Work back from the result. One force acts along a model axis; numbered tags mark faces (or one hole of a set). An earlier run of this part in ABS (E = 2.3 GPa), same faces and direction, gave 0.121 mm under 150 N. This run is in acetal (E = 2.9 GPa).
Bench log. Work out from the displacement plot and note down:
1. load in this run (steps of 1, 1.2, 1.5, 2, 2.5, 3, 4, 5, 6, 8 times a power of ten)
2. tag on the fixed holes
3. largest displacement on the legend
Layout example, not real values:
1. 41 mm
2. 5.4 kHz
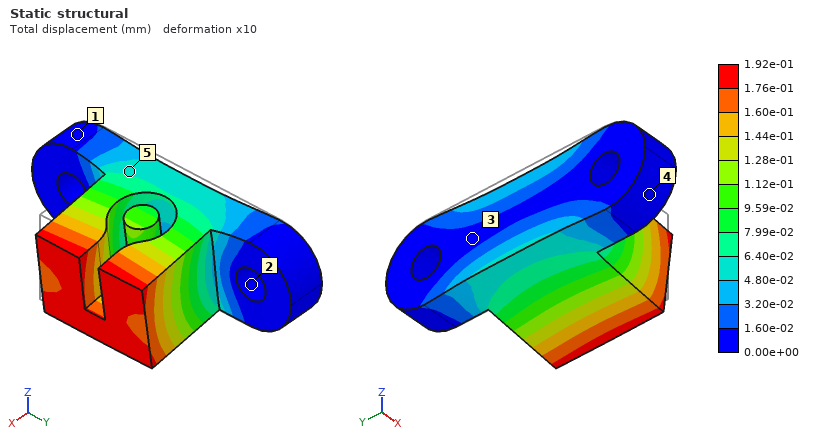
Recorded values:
1. 300 N
2. 2
3. 1.92e-01 mm
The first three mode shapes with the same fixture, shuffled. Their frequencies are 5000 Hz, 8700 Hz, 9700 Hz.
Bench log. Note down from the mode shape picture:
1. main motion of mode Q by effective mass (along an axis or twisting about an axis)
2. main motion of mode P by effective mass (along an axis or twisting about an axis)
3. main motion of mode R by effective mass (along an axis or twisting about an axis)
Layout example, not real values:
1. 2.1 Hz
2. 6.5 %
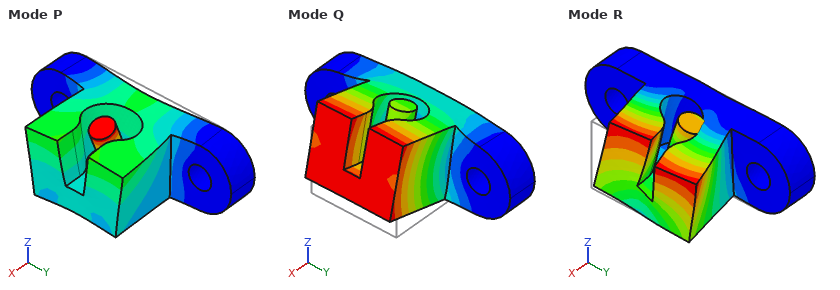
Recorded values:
1. along Z
2. along X
3. along Y
